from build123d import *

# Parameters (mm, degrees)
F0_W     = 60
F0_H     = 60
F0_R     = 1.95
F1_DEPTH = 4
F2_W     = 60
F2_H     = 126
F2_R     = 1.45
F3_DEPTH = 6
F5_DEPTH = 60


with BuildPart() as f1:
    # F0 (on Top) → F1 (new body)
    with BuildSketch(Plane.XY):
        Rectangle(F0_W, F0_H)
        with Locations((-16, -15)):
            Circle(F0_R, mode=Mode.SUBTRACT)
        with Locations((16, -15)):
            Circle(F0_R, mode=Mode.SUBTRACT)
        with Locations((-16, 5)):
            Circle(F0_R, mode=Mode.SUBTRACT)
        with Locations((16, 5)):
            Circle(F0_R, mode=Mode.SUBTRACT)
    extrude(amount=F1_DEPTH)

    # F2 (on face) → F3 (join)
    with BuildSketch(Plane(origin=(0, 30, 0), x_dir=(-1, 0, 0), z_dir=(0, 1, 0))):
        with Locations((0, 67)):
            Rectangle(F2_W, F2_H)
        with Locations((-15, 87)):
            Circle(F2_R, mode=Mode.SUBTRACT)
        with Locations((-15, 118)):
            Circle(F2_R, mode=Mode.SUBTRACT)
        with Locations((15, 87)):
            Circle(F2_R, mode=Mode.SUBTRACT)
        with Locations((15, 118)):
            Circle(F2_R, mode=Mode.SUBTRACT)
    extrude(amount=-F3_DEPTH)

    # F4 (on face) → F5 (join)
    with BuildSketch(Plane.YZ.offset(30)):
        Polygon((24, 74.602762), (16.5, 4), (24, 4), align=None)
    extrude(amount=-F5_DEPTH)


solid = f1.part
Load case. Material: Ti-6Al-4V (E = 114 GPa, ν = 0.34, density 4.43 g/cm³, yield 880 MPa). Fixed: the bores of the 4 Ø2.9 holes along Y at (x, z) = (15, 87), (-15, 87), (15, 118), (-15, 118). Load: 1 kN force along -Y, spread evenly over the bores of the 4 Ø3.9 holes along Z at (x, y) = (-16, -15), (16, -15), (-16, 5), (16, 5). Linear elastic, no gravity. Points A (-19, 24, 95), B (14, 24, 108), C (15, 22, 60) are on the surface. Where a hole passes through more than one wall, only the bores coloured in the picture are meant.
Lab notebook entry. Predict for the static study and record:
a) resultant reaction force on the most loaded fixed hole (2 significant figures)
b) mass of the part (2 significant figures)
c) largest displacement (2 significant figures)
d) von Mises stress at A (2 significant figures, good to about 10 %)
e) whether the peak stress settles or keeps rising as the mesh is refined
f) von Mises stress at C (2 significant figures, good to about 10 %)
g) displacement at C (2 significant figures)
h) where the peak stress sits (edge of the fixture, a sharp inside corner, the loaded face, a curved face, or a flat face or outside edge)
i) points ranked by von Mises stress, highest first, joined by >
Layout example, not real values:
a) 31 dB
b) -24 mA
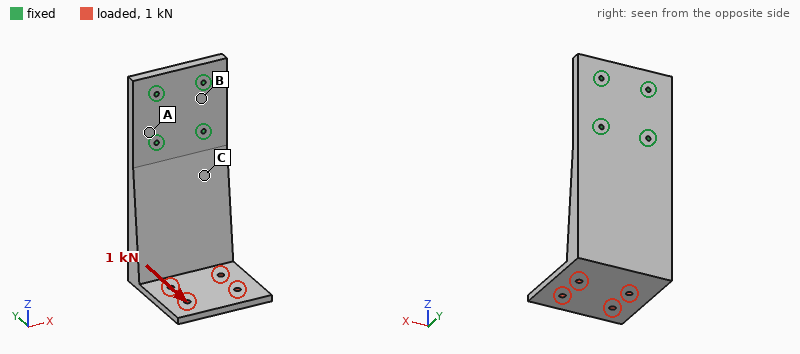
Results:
a) 1.1 kN
b) 330 g
c) 1.7 mm
d) 52 MPa
e) keeps rising
f) 94 MPa
g) 0.27 mm
h) edge of the fixture
i) C > A > B
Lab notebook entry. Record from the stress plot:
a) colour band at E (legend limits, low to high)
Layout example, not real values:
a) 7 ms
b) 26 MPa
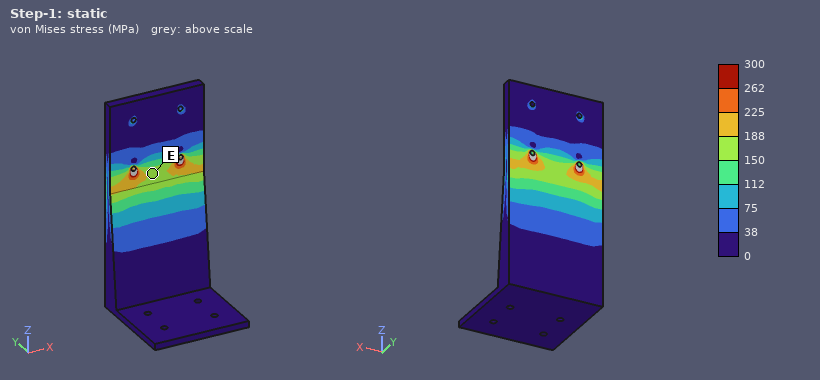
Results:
a) 150 to 188 MPa
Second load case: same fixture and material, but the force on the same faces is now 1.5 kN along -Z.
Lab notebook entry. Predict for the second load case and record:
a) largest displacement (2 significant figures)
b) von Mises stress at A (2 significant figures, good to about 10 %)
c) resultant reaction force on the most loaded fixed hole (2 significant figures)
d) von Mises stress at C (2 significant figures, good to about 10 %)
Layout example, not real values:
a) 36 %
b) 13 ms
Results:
a) 1.6 mm
b) 31 MPa
c) 700 N
d) 80 MPa
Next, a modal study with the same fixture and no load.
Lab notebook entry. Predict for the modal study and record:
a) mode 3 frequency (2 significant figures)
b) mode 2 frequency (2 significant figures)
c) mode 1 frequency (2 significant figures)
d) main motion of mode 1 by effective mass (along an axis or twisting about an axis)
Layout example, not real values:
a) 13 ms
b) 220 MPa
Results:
a) 1400 Hz
b) 1200 Hz
c) 370 Hz
d) along Y
